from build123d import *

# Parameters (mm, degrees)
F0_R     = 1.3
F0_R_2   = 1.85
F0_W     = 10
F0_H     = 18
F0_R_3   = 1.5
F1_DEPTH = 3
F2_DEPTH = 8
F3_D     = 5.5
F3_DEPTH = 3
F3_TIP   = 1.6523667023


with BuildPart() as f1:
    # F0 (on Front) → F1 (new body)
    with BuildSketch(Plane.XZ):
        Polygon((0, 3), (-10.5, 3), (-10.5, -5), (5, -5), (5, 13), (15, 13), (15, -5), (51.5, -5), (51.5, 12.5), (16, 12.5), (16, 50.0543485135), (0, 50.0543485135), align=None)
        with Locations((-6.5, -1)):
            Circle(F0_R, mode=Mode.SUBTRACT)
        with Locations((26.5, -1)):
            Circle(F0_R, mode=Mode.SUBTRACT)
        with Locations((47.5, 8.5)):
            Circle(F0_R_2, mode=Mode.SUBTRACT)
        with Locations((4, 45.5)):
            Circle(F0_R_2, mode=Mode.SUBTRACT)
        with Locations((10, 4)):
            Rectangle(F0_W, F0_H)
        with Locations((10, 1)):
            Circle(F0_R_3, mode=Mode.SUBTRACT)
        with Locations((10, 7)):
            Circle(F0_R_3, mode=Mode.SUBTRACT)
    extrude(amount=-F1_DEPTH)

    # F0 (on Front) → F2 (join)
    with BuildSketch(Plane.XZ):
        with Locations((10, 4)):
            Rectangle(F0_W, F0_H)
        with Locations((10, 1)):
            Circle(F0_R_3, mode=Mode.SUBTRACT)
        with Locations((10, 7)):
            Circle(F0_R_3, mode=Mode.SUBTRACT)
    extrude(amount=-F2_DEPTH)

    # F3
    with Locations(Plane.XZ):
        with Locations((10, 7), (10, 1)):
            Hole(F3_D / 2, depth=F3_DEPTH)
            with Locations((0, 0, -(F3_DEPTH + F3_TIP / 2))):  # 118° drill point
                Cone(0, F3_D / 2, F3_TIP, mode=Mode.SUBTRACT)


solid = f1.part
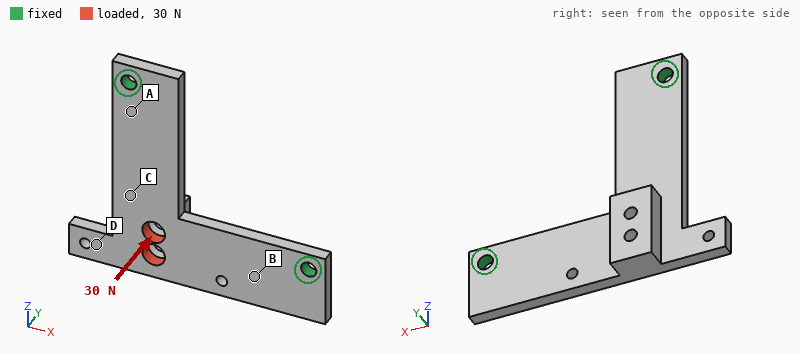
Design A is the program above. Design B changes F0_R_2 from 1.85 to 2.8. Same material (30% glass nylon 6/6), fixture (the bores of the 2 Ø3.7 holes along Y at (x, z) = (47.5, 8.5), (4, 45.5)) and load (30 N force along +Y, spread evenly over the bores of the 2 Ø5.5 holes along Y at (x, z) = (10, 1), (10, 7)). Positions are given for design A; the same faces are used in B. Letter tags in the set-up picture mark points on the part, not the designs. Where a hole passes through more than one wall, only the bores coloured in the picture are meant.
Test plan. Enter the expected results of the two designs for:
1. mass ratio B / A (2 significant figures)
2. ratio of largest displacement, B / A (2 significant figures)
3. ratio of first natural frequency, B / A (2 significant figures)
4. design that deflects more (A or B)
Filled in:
0.98
0.89
1.1
A
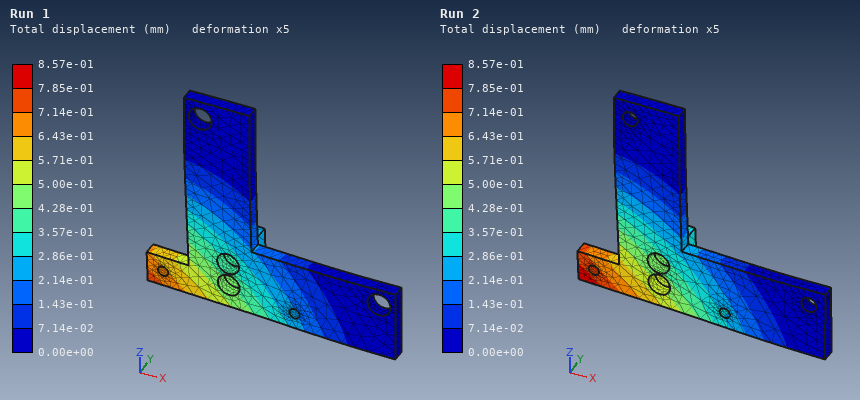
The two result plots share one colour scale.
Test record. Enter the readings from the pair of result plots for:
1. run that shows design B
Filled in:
Run 1
